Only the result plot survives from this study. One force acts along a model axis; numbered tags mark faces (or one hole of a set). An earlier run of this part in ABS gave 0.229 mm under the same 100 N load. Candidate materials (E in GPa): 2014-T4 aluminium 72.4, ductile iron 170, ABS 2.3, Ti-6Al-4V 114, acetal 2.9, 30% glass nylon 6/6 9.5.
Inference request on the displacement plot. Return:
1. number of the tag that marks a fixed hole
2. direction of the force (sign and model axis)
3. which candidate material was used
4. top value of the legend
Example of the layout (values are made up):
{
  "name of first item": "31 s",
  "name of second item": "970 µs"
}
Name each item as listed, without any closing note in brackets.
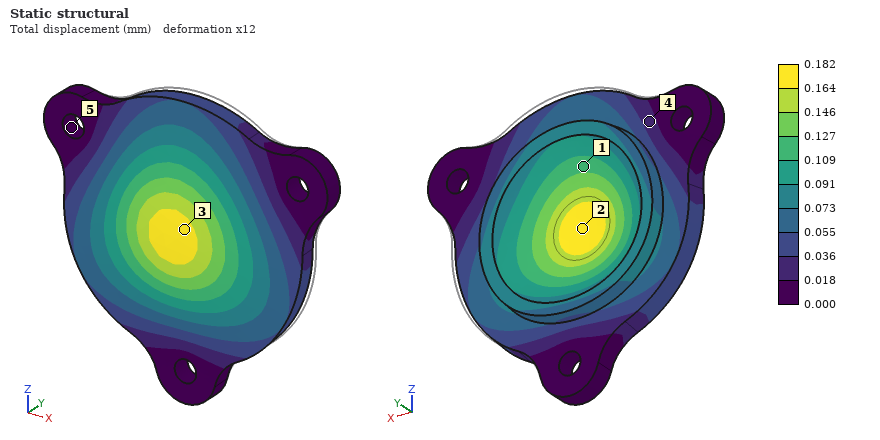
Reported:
{
  "number of the tag that marks a fixed hole": "5",
  "direction of the force": "-Y",
  "which candidate material was used": "acetal",
  "top value of the legend": "0.182 mm"
}
